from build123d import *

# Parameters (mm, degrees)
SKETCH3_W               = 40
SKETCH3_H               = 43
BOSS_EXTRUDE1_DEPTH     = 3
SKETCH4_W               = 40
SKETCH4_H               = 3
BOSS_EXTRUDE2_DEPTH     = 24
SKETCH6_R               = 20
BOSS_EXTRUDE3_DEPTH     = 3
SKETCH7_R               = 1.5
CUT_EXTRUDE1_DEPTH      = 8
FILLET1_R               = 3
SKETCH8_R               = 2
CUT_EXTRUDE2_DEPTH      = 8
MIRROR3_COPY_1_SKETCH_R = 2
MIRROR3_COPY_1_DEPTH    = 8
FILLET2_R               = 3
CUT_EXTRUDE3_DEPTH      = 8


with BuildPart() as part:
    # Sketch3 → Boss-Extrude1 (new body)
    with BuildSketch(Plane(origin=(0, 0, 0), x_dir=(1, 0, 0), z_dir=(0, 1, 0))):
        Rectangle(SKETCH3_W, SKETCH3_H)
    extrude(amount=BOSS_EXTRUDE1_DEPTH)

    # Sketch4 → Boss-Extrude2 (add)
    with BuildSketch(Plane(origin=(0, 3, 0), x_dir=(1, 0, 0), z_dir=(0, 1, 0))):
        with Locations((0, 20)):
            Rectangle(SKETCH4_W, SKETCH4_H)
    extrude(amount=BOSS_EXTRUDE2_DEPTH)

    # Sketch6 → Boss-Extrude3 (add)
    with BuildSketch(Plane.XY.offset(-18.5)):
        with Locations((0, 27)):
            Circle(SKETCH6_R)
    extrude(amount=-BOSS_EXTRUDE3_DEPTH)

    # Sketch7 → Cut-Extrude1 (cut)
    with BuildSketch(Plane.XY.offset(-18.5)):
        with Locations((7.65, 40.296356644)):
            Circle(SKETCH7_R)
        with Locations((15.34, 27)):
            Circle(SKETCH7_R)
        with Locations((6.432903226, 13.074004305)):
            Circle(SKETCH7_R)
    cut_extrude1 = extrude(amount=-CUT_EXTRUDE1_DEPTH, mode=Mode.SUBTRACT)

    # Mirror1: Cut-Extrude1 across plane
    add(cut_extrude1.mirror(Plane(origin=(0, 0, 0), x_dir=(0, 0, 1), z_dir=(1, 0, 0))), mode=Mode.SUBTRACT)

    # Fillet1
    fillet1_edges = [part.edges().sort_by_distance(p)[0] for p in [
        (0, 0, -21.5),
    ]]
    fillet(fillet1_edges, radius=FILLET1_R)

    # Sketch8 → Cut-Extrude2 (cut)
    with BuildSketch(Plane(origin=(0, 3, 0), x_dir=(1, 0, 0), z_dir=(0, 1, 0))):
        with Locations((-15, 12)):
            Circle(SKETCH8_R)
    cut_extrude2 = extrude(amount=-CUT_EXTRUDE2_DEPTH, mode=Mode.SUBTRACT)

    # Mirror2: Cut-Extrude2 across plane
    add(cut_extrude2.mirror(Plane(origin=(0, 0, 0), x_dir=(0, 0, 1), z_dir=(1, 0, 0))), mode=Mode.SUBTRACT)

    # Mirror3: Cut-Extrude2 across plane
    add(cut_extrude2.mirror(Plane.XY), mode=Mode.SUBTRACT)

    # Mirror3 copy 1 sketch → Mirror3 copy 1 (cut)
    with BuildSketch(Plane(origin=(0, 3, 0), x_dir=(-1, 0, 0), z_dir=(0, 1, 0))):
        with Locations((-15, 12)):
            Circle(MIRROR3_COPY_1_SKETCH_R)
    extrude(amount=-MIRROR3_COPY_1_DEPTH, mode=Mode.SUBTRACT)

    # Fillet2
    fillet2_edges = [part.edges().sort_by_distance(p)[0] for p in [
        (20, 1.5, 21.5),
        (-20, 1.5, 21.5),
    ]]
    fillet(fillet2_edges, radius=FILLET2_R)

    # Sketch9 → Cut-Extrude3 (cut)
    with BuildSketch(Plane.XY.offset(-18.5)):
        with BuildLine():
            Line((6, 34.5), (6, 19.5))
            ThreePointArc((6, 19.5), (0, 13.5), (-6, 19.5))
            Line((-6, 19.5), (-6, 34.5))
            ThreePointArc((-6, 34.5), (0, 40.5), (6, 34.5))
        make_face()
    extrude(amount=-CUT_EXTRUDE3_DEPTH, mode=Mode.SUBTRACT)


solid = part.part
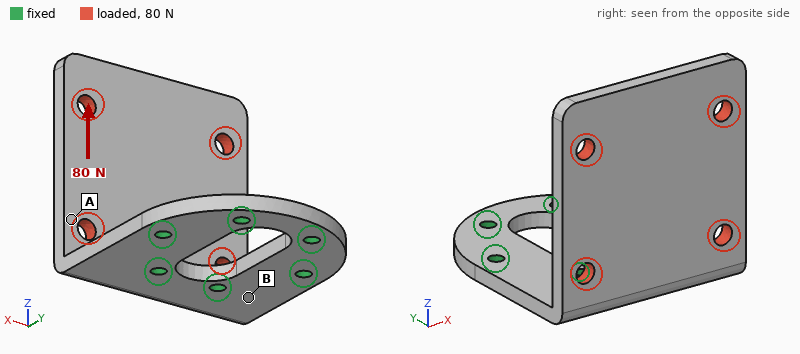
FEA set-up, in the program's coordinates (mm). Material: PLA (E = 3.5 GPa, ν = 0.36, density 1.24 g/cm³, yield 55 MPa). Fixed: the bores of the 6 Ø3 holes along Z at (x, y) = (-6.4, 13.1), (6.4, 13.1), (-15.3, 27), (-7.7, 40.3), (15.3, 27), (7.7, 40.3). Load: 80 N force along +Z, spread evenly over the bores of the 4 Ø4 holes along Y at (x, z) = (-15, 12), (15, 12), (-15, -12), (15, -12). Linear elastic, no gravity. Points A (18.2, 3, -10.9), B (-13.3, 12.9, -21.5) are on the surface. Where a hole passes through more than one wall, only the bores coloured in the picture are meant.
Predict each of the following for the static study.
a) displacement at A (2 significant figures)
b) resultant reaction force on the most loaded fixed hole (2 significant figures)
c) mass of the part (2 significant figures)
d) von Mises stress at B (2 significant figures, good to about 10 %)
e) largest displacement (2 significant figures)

0.21 mm
48 N
11 g
6.7 MPa
0.77 mm
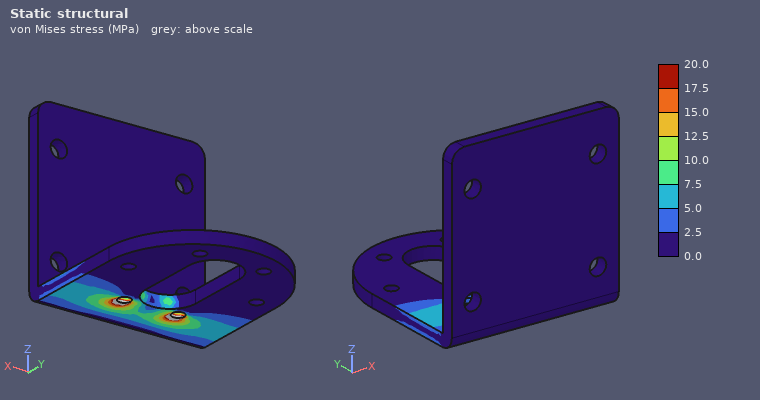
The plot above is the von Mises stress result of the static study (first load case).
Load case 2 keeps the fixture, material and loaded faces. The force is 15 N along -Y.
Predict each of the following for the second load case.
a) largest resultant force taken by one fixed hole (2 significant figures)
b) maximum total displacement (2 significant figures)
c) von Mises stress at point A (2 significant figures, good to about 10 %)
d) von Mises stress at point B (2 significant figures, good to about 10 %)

7.2 N
0.82 mm
3.6 MPa
2.7 MPa
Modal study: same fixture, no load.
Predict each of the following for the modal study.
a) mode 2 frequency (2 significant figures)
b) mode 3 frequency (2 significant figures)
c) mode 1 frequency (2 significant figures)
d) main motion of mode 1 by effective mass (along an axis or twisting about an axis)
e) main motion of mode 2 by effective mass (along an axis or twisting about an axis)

710 Hz
1100 Hz
330 Hz
along Y
along X
